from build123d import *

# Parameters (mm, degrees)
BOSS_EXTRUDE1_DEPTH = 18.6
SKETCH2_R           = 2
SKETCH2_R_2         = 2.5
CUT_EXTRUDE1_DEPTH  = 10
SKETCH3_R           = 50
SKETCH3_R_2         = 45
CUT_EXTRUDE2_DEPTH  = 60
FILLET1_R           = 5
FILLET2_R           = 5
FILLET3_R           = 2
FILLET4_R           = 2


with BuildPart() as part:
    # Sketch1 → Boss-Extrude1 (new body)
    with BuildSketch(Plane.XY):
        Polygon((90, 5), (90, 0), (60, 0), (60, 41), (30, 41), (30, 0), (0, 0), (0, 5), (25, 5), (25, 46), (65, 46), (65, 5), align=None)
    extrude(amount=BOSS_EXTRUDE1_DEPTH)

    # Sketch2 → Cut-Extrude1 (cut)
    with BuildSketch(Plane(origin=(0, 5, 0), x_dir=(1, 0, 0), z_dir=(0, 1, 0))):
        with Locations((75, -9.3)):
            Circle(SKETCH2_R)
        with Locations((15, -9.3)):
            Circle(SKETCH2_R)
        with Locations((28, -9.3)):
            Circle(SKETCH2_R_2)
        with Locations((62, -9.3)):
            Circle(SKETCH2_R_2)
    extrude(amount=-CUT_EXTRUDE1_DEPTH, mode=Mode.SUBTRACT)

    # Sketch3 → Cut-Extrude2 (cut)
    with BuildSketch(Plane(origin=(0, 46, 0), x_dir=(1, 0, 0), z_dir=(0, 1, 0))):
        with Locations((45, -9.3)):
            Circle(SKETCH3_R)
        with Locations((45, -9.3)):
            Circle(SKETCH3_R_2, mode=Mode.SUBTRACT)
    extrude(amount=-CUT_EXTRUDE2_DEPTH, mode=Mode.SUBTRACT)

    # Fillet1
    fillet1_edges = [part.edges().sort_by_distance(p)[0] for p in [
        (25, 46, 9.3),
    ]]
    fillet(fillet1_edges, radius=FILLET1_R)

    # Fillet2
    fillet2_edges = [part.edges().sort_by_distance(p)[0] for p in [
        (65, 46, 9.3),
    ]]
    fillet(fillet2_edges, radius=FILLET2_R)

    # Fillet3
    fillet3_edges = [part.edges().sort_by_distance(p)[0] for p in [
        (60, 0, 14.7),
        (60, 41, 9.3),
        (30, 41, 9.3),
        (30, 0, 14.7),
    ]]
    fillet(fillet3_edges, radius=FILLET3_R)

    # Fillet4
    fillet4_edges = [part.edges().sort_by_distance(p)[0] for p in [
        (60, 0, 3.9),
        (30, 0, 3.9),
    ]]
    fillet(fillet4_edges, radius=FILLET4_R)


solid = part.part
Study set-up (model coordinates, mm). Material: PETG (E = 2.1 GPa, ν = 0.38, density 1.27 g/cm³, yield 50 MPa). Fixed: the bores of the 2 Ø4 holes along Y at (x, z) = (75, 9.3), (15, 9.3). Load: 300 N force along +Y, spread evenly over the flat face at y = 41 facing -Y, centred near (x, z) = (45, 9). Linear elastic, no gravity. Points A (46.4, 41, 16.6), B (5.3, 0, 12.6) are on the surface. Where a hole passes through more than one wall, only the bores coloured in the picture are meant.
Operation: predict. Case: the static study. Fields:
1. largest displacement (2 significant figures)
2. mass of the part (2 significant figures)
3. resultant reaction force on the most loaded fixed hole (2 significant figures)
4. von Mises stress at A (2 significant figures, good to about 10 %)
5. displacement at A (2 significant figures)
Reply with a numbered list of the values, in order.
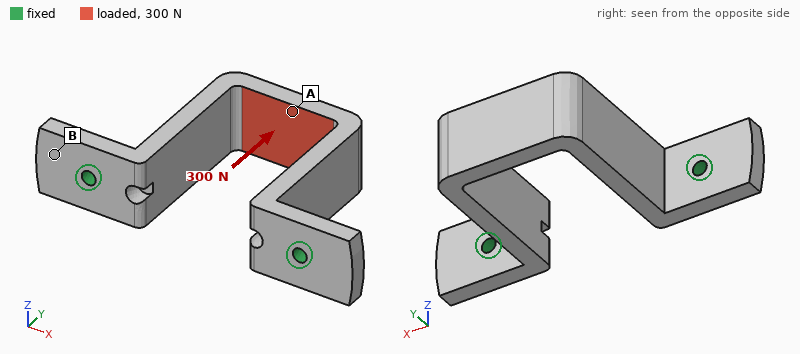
1. 0.38 mm
2. 20 g
3. 150 N
4. 9.3 MPa
5. 0.37 mm
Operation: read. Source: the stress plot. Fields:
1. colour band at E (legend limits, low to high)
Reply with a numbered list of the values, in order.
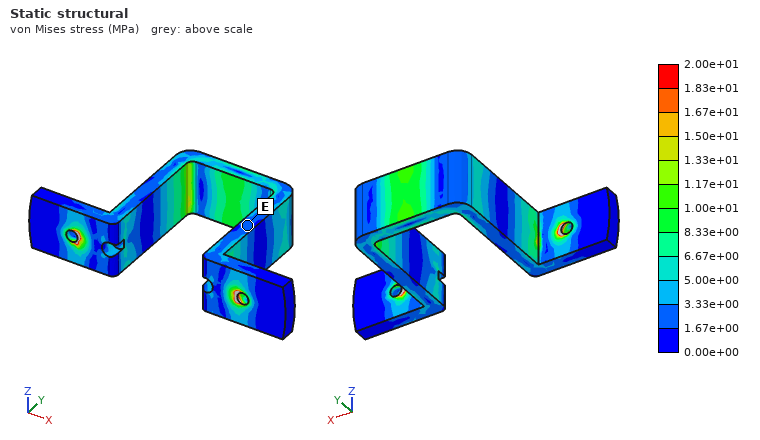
1. 1.67e+00 to 3.33e+00 MPa
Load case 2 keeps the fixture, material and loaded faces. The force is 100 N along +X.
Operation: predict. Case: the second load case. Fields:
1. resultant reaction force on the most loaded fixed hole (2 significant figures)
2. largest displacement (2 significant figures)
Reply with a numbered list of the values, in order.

1. 76 N
2. 1.1 mm
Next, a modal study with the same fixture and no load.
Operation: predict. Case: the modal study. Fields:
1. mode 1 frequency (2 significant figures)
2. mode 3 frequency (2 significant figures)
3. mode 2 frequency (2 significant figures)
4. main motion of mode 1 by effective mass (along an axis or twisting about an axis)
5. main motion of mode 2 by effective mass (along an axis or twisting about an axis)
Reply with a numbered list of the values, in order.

1. 430 Hz
2. 910 Hz
3. 550 Hz
4. along Z
5. along X
